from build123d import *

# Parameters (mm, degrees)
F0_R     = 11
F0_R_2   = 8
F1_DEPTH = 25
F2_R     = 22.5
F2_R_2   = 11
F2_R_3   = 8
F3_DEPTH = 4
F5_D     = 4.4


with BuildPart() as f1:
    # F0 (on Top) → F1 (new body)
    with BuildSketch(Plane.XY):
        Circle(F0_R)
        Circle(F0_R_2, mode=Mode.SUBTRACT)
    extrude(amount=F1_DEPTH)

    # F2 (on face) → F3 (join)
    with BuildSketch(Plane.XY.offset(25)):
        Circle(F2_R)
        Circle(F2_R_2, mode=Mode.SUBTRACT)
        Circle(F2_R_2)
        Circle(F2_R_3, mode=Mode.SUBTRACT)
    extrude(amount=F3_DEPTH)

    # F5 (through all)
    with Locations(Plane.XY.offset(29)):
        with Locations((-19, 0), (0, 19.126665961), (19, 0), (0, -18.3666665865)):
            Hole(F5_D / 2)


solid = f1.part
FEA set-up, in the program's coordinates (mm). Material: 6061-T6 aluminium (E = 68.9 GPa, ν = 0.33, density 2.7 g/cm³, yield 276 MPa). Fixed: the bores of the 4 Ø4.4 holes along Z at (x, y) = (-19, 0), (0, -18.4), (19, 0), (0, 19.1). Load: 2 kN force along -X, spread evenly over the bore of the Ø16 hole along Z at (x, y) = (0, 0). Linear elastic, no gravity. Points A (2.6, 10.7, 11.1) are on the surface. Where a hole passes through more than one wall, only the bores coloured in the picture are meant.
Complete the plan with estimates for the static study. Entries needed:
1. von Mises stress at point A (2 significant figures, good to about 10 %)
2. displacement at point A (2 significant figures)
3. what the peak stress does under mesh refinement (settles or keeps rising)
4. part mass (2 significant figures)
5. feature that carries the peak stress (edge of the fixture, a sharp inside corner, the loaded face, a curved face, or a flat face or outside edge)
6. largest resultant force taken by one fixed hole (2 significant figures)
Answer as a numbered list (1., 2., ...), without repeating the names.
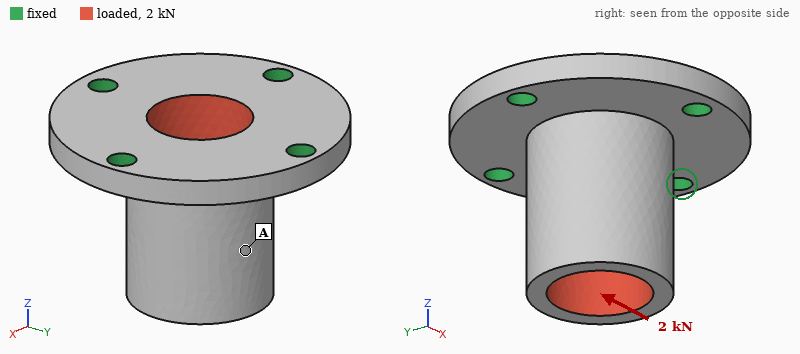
1. 13 MPa
2. 28 µm
3. keeps rising
4. 26 g
5. edge of the fixture
6. 1.0 kN
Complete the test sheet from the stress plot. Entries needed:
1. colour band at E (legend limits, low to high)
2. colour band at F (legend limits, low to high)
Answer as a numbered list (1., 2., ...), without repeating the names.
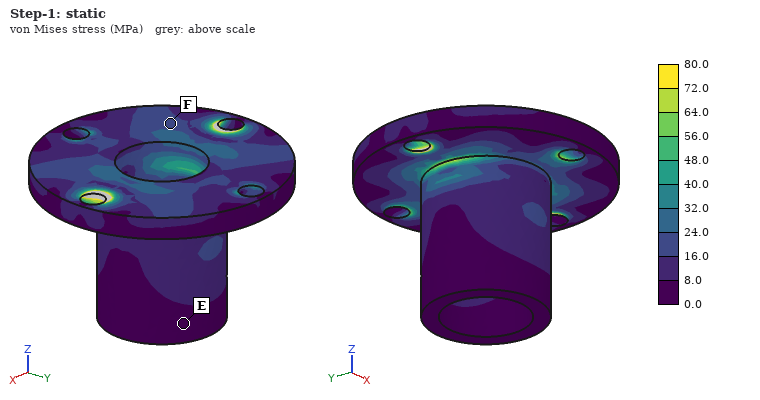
1. 0.0 to 8.0 MPa
2. 16.0 to 24.0 MPa
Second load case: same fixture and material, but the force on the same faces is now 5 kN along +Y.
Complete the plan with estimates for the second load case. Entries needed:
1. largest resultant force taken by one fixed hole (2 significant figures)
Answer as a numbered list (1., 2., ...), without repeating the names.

1. 2.6 kN
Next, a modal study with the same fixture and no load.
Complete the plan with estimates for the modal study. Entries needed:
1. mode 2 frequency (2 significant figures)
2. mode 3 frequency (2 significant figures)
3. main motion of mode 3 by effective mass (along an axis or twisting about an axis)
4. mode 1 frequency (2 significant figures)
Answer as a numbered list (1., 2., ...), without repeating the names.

1. 10000 Hz
2. 17 kHz
3. along Z
4. 9900 Hz
